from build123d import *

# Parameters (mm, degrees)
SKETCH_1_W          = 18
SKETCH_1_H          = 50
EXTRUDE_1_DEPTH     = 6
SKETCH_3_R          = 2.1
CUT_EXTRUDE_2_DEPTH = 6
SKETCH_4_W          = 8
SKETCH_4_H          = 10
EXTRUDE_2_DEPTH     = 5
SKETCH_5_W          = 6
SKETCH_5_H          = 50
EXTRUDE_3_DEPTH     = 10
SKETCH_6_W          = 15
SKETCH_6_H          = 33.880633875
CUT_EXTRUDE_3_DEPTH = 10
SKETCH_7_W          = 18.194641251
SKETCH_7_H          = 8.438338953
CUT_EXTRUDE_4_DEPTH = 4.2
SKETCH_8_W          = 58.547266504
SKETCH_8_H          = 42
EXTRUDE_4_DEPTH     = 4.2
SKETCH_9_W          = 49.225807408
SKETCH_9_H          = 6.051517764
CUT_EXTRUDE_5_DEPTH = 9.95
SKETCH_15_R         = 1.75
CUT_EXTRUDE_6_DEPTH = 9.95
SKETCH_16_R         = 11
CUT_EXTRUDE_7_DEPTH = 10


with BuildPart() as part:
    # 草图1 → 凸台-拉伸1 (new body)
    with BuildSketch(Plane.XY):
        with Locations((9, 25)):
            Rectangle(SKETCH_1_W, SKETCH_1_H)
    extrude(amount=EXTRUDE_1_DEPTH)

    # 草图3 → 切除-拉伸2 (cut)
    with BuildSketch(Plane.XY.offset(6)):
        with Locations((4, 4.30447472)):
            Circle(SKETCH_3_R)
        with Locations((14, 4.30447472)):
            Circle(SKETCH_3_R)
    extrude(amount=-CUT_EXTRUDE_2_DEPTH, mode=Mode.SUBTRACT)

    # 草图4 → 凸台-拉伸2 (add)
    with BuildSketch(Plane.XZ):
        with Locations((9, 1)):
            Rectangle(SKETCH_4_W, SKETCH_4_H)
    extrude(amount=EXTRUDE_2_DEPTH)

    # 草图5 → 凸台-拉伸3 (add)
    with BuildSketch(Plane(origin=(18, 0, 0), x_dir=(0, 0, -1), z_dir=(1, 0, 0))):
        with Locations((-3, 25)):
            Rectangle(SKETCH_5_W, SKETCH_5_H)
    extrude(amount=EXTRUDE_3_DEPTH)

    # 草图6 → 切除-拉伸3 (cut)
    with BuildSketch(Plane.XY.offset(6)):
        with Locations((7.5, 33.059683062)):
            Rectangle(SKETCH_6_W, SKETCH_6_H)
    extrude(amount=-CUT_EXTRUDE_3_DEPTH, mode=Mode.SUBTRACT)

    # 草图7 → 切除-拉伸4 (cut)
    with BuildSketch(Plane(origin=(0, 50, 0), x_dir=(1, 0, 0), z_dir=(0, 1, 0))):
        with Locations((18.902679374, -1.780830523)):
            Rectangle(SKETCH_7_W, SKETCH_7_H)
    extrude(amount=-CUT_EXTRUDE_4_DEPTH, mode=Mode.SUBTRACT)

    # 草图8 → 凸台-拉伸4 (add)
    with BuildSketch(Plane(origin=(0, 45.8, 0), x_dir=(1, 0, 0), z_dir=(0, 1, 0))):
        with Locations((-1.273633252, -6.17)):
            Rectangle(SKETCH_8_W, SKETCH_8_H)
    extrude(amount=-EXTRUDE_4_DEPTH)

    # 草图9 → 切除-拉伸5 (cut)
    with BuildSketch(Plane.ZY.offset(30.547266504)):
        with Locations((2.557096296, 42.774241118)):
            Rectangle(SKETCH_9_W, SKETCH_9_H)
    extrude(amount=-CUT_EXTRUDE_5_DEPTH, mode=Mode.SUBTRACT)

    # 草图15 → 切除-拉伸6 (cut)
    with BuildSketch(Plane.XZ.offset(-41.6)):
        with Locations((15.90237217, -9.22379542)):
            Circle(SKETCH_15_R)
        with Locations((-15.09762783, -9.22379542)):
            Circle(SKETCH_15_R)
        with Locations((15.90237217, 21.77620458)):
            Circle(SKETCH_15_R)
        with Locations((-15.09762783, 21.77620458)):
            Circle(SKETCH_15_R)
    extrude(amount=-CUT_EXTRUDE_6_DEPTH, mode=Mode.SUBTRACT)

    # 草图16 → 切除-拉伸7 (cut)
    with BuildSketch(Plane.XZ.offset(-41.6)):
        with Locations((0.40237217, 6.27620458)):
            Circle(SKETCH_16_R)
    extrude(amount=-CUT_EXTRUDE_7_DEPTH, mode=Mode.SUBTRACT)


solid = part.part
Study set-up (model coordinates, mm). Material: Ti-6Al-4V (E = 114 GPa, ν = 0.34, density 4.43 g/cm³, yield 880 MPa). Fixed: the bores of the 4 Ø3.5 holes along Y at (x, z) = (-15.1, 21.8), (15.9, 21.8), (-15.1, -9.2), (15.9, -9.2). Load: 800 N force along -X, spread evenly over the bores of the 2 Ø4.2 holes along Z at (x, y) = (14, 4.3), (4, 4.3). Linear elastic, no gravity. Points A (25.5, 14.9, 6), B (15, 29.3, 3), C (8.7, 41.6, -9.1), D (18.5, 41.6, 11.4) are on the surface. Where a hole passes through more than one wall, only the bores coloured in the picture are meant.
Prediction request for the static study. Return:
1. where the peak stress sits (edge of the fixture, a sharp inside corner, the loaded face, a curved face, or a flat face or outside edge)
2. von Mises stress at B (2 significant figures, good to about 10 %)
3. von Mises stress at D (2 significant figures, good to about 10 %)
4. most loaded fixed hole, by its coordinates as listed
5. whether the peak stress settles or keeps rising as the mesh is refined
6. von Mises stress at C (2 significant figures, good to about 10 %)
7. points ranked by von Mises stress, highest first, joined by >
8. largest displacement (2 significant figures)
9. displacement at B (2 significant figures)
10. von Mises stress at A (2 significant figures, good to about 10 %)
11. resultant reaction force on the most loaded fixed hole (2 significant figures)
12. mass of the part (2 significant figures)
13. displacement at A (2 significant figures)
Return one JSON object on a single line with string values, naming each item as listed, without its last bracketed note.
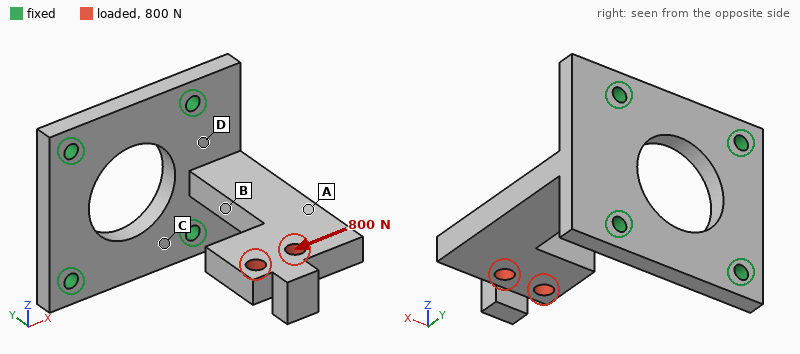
{"where the peak stress sits": "edge of the fixture", "von Mises stress at B": "120 MPa", "von Mises stress at D": "190 MPa", "most loaded fixed hole, by its coordinates as listed": "(15.9, -9.2)", "whether the peak stress settles or keeps rising as the mesh is refined": "keeps rising", "von Mises stress at C": "73 MPa", "points ranked by von Mises stress, highest first, joined by >": "D > B > C > A", "largest displacement": "0.73 mm", "displacement at B": "0.18 mm", "von Mises stress at A": "35 MPa", "resultant reaction force on the most loaded fixed hole": "490 N", "mass of the part": "52 g", "displacement at A": "0.40 mm"}
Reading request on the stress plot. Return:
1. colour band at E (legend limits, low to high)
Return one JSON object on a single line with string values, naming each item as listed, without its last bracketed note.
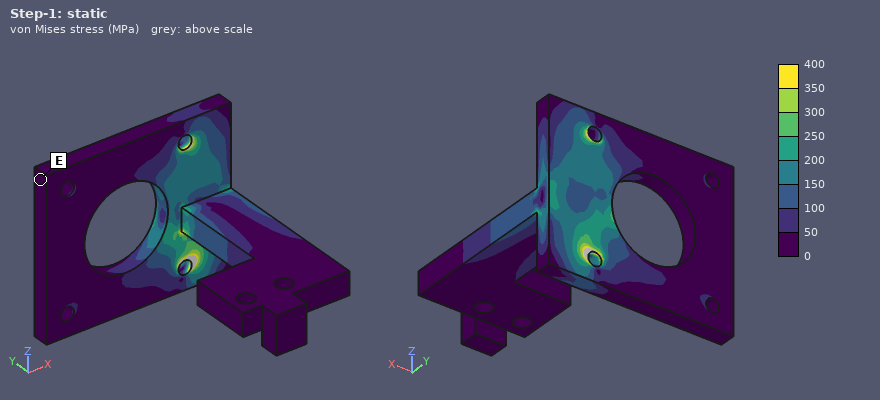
{"colour band at E": "0 to 50 MPa"}
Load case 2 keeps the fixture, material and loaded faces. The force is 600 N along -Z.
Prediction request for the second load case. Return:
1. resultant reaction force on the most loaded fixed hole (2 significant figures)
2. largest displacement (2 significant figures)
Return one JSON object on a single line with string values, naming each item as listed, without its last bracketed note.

{"resultant reaction force on the most loaded fixed hole": "1.1 kN", "largest displacement": "0.90 mm"}
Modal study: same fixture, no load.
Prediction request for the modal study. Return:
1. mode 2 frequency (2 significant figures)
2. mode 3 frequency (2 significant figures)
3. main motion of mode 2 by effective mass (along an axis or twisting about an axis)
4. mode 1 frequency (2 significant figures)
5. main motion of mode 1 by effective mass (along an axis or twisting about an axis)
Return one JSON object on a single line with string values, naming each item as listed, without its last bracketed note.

{"mode 2 frequency": "1600 Hz", "mode 3 frequency": "5000 Hz", "main motion of mode 2 by effective mass": "along X", "mode 1 frequency": "1400 Hz", "main motion of mode 1 by effective mass": "along Z"}
